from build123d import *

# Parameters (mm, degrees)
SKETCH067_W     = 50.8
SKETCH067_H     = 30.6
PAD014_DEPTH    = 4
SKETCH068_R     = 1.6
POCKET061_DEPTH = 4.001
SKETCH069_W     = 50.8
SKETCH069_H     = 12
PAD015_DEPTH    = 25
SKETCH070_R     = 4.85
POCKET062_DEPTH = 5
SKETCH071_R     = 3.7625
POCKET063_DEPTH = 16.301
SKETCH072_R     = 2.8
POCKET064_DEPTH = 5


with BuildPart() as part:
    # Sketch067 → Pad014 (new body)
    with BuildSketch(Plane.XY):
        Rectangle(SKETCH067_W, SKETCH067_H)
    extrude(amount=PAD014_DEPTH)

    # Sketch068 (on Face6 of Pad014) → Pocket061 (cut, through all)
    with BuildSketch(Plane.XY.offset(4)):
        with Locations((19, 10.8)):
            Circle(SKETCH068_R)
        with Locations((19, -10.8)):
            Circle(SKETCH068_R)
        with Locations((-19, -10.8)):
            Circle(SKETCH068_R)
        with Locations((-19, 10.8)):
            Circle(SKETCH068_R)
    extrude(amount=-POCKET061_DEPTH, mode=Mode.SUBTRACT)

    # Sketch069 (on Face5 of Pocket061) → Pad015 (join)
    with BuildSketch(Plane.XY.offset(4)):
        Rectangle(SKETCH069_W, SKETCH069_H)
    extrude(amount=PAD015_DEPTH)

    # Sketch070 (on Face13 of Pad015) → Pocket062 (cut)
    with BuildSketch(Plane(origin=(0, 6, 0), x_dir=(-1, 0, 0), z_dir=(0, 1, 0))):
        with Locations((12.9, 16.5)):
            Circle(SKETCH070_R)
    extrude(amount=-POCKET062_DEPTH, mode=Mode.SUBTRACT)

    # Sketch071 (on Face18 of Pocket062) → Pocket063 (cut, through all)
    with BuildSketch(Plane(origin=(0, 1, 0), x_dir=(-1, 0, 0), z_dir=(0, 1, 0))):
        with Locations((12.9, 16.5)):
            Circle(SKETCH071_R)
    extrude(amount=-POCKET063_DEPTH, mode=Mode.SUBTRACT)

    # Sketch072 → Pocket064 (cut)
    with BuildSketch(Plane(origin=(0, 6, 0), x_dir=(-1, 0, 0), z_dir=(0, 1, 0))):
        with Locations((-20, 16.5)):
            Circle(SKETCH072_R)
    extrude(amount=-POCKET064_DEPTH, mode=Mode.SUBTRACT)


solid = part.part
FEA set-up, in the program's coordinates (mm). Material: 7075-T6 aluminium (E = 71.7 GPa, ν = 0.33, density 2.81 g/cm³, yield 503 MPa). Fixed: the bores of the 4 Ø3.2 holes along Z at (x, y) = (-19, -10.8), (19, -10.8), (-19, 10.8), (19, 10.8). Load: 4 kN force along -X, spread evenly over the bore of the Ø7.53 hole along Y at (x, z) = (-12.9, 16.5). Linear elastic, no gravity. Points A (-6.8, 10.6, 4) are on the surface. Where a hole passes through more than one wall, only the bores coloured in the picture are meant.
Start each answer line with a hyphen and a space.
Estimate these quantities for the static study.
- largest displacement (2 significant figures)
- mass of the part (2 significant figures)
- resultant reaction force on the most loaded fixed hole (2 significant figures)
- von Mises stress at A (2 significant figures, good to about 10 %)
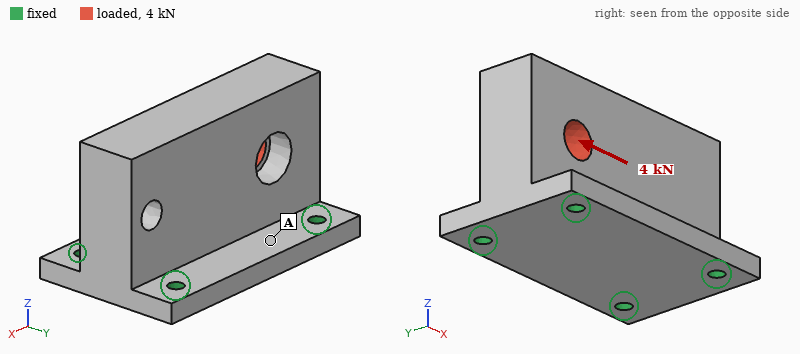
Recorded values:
- 25 µm
- 58 g
- 1.4 kN
- 16 MPa
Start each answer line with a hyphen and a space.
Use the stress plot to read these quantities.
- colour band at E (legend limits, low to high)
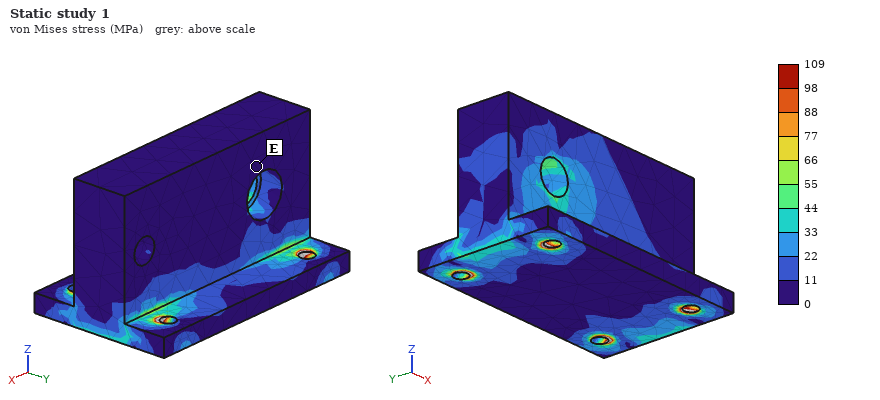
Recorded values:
- 0 to 11 MPa
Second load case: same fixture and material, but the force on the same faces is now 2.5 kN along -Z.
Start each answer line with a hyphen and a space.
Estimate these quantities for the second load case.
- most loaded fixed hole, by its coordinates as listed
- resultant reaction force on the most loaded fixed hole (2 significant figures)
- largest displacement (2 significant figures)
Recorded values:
- (-19, -10.8)
- 1.3 kN
- 19 µm
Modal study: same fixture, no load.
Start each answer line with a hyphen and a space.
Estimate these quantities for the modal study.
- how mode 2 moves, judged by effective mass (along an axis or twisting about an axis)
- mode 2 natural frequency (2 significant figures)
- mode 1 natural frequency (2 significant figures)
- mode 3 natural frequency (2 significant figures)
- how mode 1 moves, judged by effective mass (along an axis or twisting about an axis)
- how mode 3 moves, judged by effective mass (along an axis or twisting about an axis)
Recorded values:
- along X
- 11 kHz
- 6900 Hz
- 13 kHz
- along Y
- along Z
